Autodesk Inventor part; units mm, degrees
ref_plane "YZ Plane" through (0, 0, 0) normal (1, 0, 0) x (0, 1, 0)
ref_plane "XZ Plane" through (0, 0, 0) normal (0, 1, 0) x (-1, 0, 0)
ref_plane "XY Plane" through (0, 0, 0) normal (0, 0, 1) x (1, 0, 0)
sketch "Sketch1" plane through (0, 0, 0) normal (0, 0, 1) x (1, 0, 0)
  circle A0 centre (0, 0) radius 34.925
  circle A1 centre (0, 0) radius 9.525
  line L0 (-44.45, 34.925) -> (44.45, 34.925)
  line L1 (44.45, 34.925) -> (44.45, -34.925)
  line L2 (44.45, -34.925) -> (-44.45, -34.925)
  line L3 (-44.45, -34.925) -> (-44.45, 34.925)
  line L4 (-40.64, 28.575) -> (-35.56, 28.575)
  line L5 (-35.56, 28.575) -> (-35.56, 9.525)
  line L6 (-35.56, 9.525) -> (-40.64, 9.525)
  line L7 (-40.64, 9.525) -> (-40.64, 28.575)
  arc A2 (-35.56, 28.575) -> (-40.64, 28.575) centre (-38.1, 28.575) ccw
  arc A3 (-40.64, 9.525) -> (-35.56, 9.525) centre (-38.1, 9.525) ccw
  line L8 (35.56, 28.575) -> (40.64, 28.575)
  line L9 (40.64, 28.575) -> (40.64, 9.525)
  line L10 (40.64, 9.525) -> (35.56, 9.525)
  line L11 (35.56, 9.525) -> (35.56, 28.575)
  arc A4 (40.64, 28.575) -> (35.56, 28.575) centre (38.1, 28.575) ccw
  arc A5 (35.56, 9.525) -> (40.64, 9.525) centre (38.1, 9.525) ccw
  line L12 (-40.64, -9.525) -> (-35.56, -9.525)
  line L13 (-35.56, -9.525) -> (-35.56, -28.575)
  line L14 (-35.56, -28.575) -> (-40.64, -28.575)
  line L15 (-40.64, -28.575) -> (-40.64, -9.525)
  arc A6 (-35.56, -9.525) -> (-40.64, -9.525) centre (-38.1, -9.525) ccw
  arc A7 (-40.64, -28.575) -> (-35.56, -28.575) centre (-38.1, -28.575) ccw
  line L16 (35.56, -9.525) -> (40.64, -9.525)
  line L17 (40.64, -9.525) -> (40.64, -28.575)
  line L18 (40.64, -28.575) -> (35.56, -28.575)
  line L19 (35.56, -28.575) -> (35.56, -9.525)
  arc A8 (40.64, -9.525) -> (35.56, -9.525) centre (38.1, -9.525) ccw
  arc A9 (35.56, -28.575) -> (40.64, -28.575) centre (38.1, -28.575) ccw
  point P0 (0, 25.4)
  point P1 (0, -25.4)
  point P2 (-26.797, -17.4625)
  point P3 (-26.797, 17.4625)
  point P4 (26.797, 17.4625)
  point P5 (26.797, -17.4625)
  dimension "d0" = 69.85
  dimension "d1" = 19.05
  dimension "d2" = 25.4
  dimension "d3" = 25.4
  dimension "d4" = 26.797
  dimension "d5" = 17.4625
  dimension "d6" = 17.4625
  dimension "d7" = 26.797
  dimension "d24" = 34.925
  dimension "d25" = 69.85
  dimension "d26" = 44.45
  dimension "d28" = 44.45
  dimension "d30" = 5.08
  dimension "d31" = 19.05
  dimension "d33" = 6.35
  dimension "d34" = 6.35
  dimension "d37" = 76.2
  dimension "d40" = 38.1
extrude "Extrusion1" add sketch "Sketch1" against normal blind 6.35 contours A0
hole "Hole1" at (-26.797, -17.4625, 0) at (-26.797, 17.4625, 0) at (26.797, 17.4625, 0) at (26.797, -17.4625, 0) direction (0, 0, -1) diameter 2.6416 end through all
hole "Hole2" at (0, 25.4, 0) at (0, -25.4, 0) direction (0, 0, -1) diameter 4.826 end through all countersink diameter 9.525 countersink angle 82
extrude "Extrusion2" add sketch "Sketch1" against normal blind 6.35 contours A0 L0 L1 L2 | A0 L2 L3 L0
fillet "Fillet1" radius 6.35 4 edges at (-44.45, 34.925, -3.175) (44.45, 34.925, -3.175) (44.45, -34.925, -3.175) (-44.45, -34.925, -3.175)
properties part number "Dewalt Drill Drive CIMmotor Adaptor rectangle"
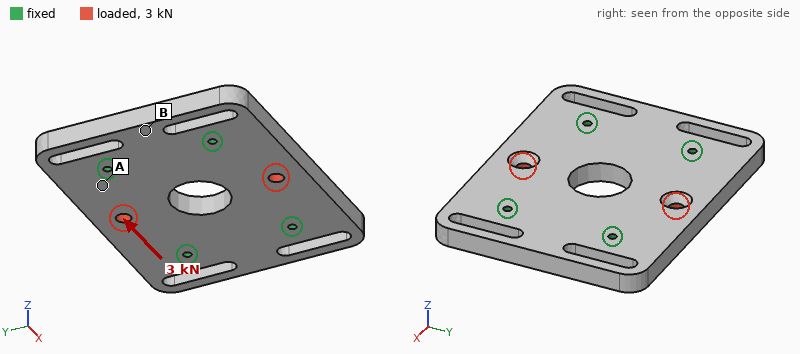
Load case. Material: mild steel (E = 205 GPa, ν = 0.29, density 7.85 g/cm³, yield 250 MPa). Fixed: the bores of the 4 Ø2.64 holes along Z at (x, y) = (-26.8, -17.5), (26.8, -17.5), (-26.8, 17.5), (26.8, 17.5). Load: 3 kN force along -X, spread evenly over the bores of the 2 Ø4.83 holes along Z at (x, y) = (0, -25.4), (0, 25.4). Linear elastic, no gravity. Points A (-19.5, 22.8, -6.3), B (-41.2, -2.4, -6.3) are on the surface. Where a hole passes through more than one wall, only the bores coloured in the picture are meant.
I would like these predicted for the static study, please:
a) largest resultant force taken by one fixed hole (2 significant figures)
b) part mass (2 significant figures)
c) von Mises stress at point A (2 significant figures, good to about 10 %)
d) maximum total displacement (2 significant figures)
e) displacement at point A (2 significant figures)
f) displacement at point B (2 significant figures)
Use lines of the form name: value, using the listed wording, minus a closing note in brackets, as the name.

largest resultant force taken by one fixed hole: 760 N
part mass: 270 g
von Mises stress at point A: 7.5 MPa
maximum total displacement: 1.7 µm
displacement at point A: 0.49 µm
displacement at point B: 0.29 µm
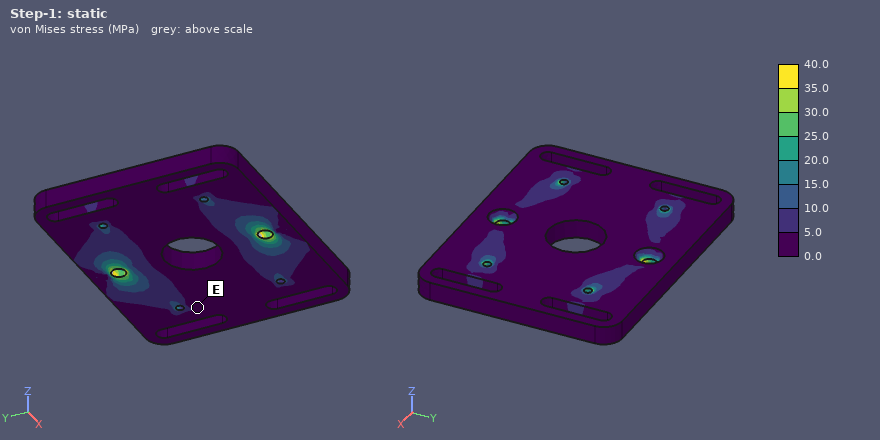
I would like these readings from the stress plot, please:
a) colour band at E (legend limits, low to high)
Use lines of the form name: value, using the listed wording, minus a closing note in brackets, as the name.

colour band at E: 0.0 to 5.0 MPa
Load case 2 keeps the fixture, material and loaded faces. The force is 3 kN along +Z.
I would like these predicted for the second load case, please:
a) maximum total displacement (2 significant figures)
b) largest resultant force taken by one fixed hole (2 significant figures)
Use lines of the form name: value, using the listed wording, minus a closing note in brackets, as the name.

maximum total displacement: 28 µm
largest resultant force taken by one fixed hole: 750 N
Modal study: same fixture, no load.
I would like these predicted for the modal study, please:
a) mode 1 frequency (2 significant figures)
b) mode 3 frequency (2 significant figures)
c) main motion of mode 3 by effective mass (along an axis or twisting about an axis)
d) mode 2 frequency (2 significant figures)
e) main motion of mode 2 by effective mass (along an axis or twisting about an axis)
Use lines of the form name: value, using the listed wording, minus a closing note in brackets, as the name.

mode 1 frequency: 7200 Hz
mode 3 frequency: 9500 Hz
main motion of mode 3 by effective mass: along Z
mode 2 frequency: 8100 Hz
main motion of mode 2 by effective mass: twisting about X
